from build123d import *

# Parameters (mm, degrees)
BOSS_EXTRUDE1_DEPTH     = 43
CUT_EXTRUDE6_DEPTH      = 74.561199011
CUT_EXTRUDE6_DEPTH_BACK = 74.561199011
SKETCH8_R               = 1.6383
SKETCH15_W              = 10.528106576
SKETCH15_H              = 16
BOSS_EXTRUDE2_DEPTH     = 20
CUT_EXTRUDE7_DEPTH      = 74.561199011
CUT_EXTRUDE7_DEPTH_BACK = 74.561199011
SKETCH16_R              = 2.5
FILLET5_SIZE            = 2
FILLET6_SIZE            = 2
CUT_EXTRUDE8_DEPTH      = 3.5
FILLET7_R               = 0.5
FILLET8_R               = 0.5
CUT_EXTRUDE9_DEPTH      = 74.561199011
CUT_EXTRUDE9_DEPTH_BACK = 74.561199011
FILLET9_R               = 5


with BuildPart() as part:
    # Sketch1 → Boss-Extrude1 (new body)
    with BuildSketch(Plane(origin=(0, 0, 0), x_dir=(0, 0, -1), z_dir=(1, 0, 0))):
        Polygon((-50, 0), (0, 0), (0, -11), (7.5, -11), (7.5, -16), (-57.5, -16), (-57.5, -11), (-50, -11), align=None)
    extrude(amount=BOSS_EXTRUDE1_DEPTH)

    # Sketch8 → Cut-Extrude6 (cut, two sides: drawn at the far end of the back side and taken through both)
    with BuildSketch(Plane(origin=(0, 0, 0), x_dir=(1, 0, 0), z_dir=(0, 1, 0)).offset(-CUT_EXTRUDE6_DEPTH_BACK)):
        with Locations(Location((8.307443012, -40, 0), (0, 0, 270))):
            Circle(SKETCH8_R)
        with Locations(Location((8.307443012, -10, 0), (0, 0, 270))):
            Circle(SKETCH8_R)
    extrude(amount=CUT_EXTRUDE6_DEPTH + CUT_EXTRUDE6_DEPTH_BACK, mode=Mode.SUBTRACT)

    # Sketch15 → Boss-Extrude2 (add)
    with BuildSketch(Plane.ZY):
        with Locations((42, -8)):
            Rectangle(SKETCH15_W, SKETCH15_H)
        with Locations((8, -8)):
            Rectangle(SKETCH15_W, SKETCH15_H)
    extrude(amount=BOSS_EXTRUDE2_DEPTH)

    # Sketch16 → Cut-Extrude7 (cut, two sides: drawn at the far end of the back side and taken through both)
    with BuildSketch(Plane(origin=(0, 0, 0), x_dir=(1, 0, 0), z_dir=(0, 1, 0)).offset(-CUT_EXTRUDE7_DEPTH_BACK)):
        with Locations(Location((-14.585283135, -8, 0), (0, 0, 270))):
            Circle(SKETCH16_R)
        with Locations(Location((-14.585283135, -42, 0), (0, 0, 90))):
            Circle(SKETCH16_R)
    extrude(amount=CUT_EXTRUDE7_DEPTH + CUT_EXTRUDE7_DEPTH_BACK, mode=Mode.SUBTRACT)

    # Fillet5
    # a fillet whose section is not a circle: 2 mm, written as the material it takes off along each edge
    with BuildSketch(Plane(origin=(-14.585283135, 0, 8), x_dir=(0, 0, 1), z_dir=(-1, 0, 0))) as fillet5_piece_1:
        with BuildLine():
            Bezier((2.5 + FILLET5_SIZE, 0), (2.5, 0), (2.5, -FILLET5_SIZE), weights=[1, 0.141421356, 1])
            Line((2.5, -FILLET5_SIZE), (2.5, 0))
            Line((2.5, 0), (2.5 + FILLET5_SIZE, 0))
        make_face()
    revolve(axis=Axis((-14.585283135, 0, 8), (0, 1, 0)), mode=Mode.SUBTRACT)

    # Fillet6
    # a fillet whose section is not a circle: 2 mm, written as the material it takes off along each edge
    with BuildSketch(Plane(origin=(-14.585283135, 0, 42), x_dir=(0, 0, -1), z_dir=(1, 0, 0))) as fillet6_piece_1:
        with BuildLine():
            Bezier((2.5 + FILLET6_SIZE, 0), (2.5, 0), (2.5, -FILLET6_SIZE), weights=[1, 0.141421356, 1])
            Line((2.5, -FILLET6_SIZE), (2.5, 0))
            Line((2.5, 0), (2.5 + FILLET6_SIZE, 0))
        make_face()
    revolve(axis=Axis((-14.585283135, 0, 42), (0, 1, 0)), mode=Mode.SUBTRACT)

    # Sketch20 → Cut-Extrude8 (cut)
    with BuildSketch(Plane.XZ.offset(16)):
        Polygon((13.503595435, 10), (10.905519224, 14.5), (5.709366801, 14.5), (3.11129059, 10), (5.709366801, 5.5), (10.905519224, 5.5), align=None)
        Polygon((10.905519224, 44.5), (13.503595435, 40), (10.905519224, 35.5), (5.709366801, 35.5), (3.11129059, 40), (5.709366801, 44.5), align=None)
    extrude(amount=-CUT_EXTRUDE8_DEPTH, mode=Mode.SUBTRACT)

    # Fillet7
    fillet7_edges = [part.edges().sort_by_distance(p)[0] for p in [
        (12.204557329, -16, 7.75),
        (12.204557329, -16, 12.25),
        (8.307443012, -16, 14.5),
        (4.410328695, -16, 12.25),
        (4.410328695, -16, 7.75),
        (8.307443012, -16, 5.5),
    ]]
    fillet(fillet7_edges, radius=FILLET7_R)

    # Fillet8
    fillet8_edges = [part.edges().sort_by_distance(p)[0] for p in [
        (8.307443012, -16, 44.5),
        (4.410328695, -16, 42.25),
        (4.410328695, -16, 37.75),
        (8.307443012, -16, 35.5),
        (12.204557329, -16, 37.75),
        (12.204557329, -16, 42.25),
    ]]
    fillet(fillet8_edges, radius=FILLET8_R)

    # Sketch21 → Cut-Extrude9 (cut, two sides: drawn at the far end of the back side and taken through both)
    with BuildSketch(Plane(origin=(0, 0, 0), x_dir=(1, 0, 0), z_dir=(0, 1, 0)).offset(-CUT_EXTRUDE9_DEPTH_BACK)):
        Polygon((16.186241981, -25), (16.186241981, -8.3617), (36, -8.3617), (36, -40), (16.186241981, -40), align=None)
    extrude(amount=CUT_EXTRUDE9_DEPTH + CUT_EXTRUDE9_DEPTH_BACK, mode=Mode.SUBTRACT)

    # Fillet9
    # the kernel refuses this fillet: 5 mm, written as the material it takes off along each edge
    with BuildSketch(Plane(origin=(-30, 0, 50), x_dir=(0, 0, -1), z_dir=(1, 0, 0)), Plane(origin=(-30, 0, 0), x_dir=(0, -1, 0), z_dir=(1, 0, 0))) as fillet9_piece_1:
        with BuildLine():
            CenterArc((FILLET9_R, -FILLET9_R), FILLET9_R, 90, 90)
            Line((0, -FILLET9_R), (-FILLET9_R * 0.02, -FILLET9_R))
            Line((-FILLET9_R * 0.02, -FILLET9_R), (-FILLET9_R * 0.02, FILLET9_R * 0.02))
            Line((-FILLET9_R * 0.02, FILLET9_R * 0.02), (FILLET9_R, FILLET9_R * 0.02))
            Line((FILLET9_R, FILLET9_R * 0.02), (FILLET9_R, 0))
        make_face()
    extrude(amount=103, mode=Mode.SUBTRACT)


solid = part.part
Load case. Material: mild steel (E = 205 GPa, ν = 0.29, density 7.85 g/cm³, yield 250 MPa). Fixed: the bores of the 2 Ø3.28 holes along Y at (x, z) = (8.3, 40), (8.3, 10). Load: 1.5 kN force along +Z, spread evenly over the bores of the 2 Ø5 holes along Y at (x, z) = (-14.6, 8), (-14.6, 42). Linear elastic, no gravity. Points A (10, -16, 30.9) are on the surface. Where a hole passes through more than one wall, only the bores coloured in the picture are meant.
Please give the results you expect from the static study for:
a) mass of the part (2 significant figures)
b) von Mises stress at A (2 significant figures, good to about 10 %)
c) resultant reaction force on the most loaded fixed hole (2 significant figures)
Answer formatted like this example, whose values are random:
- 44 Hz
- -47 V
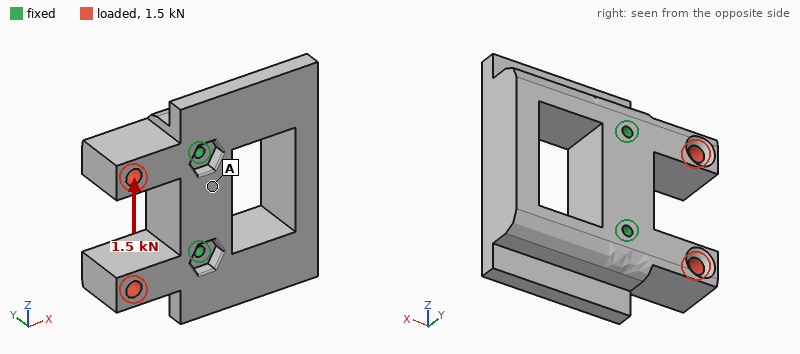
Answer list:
- 250 g
- 8.3 MPa
- 1.2 kN
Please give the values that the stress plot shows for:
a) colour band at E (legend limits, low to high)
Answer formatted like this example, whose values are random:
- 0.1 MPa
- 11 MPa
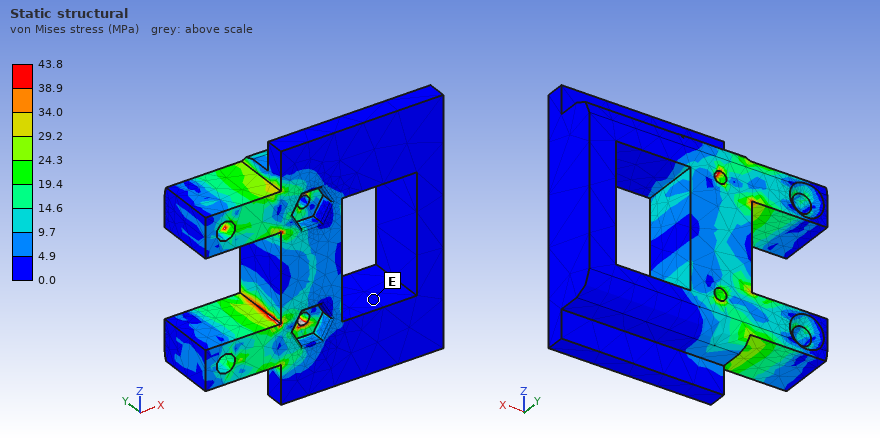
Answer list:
- 0.0 to 4.9 MPa
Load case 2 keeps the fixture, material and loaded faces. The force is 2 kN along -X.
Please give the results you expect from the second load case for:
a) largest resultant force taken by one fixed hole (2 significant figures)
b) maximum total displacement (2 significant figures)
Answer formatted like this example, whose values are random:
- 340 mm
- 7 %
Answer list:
- 1.0 kN
- 2.0 µm
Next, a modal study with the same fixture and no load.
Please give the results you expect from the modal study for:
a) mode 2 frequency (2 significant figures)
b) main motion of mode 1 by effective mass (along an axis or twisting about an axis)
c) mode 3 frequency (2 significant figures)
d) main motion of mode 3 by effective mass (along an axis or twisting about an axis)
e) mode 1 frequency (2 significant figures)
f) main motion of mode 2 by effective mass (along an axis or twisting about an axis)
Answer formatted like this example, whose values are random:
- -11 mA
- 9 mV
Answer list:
- 6200 Hz
- along Y
- 7900 Hz
- twisting about X
- 5400 Hz
- along Z
